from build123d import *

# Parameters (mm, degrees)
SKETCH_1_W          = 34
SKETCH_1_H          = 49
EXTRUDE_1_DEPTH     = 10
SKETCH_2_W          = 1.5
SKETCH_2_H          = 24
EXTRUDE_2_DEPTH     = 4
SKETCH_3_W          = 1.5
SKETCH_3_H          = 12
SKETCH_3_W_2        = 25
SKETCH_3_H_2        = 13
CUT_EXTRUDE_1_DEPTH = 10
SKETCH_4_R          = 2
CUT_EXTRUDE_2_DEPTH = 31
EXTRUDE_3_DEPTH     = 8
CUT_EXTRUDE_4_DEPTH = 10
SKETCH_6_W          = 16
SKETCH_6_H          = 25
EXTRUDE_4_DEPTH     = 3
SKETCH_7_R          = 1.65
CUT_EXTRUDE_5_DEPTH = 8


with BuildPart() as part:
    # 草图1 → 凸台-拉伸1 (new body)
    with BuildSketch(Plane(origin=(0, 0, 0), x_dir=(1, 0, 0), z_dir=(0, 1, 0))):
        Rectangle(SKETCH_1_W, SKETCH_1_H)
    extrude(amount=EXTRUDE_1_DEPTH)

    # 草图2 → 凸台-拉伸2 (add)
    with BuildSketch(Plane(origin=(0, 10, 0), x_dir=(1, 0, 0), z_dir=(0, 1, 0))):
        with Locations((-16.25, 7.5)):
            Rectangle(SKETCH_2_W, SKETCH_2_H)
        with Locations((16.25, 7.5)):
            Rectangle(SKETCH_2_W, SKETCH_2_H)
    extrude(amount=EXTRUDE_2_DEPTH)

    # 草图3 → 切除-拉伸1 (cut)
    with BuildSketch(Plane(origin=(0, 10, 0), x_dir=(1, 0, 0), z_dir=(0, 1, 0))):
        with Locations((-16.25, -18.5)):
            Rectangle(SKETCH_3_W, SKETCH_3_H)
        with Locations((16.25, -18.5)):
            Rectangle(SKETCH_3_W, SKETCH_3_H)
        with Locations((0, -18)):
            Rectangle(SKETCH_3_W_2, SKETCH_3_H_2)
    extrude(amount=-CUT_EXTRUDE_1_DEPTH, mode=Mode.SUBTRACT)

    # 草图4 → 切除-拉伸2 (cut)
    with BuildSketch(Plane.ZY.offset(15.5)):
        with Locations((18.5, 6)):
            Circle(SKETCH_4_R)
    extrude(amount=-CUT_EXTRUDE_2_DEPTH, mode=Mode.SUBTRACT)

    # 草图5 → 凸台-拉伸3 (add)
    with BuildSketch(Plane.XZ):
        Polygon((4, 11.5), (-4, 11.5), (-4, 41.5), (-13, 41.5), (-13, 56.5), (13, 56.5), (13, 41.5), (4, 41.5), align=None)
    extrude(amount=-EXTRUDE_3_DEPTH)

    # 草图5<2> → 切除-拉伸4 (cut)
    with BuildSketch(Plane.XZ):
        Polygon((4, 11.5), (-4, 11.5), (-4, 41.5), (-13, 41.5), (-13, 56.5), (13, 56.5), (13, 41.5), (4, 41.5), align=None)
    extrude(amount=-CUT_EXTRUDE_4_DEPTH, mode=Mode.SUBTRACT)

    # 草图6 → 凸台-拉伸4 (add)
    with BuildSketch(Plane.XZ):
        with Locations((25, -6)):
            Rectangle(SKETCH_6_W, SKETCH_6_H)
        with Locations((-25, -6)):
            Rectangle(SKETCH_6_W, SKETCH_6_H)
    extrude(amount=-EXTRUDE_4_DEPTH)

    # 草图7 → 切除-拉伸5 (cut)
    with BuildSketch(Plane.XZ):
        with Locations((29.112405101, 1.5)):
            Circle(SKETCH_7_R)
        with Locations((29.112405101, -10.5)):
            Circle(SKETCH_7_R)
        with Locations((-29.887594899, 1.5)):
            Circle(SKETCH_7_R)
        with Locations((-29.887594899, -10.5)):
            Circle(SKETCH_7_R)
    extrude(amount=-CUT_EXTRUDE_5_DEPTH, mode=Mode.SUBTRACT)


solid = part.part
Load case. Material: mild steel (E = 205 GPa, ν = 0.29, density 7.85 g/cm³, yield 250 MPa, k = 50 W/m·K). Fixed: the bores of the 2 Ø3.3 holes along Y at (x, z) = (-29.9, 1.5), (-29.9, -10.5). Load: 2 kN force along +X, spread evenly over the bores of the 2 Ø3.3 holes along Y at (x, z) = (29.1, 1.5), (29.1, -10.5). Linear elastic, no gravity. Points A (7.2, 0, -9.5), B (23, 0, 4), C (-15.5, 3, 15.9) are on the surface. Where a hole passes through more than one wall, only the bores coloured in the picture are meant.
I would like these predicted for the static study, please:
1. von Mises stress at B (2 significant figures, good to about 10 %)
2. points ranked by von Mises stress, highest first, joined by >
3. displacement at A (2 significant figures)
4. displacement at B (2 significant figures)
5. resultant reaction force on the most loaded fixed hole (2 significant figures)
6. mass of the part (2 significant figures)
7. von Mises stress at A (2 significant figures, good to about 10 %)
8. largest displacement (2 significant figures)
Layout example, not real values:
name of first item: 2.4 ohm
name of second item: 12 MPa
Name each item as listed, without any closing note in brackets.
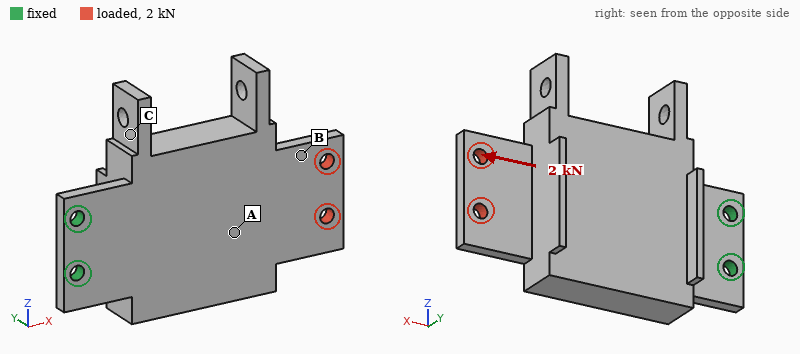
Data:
von Mises stress at B: 34 MPa
points ranked by von Mises stress, highest first, joined by >: B > A > C
displacement at A: 7.0 µm
displacement at B: 15 µm
resultant reaction force on the most loaded fixed hole: 1.0 kN
mass of the part: 120 g
von Mises stress at A: 21 MPa
largest displacement: 21 µm
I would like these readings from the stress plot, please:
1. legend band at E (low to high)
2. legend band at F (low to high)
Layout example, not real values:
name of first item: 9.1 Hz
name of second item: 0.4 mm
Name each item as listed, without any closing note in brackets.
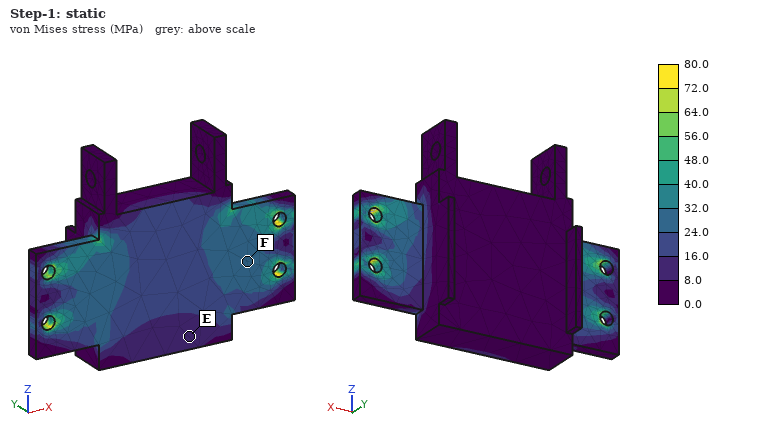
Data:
legend band at E: 8.0 to 16.0 MPa
legend band at F: 24.0 to 32.0 MPa
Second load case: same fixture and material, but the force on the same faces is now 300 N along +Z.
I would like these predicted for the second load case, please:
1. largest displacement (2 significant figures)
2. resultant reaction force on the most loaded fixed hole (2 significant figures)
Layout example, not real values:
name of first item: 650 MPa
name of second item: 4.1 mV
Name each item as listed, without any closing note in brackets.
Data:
largest displacement: 31 µm
resultant reaction force on the most loaded fixed hole: 1.2 kN
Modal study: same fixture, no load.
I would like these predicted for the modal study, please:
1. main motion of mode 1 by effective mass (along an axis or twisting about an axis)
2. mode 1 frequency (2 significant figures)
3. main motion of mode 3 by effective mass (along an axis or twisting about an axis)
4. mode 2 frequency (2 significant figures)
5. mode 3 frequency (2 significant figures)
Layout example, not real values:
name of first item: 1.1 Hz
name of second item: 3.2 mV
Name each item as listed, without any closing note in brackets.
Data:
main motion of mode 1 by effective mass: along Y
mode 1 frequency: 500 Hz
main motion of mode 3 by effective mass: along Z
mode 2 frequency: 2100 Hz
mode 3 frequency: 2800 Hz
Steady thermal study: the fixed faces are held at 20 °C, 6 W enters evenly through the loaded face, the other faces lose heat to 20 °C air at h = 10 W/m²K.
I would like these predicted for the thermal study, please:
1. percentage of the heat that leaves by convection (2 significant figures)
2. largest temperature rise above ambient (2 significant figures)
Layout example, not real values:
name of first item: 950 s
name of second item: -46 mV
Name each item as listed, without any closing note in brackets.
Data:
percentage of the heat that leaves by convection: 25 %
largest temperature rise above ambient: 54 K
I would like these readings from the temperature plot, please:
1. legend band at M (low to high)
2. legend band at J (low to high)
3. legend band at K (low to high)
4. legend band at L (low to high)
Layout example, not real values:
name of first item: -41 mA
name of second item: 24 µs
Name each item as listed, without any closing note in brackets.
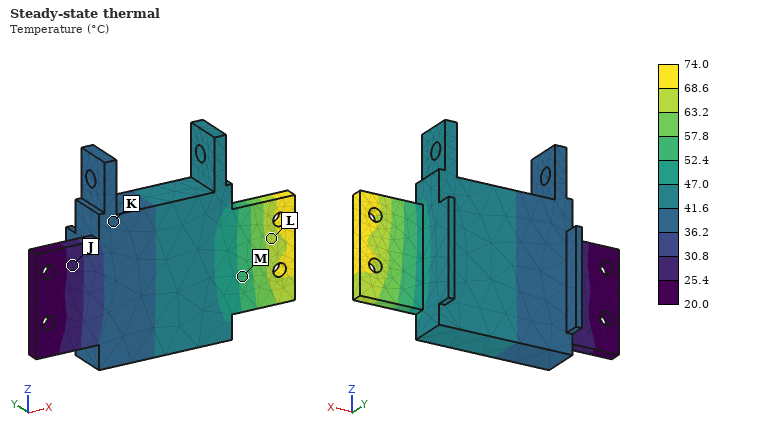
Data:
legend band at M: 52.4 to 57.8 °C
legend band at J: 25.4 to 30.8 °C
legend band at K: 36.2 to 41.6 °C
legend band at L: 63.2 to 68.6 °C
